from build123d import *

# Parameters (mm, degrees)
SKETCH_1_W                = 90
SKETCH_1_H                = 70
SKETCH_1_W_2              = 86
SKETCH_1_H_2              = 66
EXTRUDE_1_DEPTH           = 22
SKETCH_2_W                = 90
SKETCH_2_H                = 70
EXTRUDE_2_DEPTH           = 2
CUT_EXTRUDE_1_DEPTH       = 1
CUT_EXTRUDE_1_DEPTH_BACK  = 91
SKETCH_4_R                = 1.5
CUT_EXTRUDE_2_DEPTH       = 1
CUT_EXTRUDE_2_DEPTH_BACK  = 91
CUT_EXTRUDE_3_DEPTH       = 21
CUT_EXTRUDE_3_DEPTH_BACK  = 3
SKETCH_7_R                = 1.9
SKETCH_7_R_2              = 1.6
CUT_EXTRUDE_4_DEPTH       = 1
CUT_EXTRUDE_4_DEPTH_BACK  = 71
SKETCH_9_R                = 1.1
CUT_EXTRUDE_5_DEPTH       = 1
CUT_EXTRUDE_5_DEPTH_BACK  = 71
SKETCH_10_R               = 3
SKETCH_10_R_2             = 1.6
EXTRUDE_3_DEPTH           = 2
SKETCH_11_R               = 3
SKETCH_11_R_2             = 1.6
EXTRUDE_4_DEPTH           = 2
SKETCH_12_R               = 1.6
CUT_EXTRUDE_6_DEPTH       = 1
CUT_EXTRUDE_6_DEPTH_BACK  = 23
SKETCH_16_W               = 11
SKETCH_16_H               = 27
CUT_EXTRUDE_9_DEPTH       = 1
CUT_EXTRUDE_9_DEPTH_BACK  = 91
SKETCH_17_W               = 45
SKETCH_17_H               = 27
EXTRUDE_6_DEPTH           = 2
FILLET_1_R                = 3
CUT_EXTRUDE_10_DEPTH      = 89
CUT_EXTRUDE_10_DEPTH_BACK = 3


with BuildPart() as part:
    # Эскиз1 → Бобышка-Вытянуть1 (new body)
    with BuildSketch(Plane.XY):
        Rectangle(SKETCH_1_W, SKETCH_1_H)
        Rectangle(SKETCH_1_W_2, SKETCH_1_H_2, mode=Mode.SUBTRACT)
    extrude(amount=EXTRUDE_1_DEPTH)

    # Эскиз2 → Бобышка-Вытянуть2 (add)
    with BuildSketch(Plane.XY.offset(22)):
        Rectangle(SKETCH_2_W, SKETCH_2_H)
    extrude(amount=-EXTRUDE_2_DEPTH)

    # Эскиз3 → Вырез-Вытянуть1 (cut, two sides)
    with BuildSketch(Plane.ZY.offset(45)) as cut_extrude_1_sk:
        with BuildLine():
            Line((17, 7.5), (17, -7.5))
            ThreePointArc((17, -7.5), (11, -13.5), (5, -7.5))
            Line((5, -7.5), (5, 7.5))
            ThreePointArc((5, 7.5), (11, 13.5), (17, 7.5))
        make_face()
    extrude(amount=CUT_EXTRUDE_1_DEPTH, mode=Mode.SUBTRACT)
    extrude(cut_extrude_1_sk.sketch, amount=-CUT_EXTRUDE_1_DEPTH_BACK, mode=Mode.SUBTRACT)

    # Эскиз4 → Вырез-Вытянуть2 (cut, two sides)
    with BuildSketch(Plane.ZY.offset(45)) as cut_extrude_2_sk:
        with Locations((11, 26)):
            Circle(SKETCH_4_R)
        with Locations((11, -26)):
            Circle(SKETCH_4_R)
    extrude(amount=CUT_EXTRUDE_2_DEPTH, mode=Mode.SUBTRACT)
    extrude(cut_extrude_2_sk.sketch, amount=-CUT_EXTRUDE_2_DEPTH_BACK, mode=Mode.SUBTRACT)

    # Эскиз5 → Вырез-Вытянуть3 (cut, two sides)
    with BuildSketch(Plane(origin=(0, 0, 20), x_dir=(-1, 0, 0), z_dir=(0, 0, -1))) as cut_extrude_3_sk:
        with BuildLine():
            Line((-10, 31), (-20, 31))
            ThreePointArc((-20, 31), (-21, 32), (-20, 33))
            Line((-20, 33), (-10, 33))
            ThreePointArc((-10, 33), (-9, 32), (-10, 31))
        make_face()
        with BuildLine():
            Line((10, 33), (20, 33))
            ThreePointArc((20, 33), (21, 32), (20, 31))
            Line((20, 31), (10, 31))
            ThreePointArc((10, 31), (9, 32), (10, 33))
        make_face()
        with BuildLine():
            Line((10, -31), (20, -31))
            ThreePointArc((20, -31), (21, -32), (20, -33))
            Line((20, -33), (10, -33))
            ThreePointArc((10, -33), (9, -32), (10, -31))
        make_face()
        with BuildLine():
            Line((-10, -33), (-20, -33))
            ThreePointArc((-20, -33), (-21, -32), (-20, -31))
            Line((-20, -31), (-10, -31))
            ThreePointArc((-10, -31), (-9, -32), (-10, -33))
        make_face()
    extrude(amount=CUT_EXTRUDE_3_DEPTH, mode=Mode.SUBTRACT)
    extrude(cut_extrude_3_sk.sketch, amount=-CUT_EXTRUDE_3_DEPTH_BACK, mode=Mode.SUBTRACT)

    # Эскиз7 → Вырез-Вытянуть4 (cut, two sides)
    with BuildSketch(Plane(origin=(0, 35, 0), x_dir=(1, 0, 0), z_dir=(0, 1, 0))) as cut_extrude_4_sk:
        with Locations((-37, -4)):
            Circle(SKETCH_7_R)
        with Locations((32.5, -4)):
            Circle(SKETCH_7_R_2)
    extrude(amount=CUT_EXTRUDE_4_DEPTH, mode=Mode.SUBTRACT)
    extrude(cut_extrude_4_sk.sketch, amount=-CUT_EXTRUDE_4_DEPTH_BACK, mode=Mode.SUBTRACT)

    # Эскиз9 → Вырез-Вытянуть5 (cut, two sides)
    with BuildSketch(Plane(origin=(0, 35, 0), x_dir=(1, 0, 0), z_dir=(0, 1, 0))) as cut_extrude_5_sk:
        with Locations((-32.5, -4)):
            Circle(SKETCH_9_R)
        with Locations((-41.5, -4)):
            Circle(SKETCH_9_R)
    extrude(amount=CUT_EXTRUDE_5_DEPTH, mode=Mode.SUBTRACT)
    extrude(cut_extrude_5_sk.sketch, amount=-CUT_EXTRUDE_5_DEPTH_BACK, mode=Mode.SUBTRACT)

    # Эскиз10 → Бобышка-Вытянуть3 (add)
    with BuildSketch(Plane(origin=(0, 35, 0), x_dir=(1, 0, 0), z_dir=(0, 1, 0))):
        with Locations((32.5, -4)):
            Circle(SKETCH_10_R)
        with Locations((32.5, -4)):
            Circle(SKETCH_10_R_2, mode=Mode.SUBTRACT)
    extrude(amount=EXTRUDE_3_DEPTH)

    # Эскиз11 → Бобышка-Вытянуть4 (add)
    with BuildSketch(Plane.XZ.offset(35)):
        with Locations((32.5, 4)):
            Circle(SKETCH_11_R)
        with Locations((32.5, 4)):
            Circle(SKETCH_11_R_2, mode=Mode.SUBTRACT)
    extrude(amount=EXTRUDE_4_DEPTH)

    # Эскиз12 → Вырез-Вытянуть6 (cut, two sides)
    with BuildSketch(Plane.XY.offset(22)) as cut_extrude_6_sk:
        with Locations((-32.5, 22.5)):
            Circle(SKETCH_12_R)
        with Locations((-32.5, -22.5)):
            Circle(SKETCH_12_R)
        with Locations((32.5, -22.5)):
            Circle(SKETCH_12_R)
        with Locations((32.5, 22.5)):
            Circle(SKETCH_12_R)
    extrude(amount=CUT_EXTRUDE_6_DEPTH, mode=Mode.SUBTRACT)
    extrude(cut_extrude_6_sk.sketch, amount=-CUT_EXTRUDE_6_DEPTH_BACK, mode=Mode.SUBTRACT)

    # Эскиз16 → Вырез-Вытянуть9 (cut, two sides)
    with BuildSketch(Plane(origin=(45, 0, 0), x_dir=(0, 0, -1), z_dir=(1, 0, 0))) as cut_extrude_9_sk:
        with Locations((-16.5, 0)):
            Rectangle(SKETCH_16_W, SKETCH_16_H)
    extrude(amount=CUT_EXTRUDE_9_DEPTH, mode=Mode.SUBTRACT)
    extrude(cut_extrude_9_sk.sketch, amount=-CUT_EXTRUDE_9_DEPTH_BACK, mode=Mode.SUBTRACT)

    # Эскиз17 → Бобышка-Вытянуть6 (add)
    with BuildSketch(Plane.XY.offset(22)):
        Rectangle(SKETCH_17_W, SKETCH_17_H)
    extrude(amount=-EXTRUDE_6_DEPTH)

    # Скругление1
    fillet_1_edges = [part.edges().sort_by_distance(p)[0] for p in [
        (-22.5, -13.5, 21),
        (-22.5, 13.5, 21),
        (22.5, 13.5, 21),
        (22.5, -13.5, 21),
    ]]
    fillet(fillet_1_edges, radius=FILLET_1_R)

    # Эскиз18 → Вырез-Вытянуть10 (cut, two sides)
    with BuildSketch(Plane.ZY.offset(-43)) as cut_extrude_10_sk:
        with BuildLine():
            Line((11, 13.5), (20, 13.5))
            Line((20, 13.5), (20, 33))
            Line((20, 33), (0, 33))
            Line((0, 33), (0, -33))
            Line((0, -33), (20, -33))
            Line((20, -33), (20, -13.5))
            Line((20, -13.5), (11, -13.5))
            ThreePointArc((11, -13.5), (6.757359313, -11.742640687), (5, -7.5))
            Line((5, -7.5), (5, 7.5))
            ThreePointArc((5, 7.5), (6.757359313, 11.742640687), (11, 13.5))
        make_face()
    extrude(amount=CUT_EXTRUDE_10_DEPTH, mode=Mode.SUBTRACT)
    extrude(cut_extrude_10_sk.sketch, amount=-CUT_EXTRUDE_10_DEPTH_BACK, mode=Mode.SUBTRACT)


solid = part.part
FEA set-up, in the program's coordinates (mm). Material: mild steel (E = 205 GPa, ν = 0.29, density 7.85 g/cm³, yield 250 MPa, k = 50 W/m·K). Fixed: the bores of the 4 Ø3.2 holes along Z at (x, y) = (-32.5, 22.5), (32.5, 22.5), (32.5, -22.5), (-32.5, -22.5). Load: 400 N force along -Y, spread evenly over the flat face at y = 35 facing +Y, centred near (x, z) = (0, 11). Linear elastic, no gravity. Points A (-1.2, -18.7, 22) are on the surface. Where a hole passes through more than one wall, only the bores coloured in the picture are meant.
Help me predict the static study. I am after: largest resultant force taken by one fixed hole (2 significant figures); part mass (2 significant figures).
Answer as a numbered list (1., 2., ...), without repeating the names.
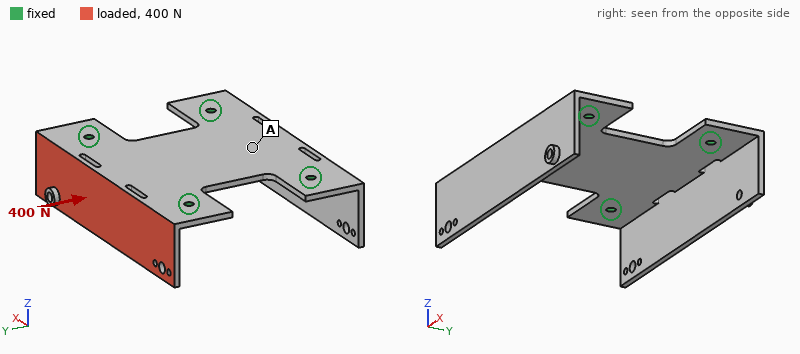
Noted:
1. 150 N
2. 130 g
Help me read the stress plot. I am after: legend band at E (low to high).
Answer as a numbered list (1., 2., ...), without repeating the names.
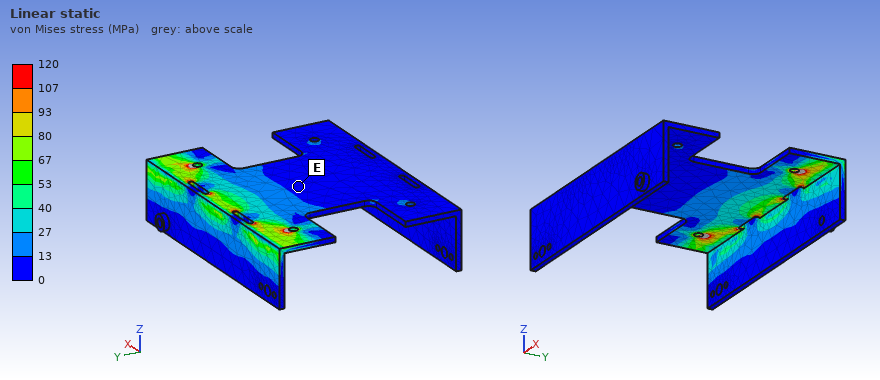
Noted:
1. 0 to 13 MPa
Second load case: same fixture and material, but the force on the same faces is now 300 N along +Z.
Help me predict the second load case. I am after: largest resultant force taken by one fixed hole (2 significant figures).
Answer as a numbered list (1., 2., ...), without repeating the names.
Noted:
1. 160 N
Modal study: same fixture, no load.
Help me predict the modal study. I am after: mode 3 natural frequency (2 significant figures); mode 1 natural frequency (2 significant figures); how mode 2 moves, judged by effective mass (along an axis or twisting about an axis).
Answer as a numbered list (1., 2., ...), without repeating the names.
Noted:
1. 2500 Hz
2. 1600 Hz
3. along Y
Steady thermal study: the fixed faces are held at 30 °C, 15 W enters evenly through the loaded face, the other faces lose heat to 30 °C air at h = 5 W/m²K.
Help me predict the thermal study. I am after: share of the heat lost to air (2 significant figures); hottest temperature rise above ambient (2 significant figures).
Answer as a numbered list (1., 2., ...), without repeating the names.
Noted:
1. 8.4 %
2. 58 K
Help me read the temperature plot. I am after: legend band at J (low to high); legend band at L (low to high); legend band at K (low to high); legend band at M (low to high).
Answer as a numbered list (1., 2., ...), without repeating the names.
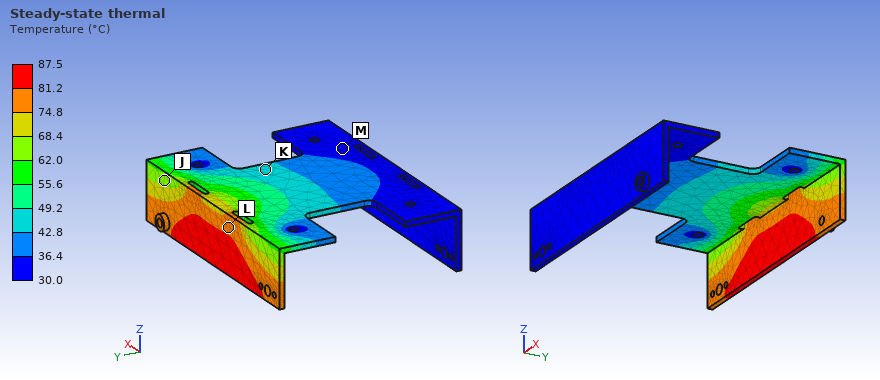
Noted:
1. 62.0 to 68.4 °C
2. 74.8 to 81.2 °C
3. 42.8 to 49.2 °C
4. 30.0 to 36.4 °C
